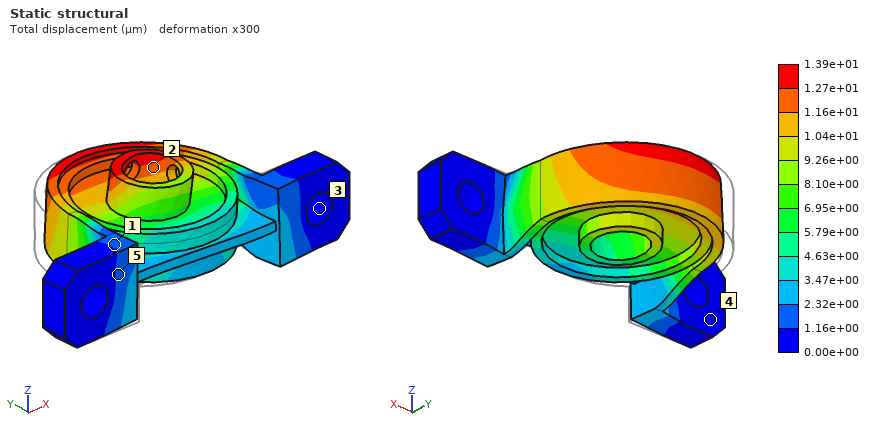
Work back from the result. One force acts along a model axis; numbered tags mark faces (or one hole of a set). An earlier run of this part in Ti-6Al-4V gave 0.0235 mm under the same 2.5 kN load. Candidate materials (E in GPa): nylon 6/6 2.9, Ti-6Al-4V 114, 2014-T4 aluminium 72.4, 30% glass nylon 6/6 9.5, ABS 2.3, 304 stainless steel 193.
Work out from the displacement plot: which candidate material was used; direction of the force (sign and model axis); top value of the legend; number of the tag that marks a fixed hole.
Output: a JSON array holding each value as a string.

["304 stainless steel", "+X", "1.39e+01 µm", "3"]
